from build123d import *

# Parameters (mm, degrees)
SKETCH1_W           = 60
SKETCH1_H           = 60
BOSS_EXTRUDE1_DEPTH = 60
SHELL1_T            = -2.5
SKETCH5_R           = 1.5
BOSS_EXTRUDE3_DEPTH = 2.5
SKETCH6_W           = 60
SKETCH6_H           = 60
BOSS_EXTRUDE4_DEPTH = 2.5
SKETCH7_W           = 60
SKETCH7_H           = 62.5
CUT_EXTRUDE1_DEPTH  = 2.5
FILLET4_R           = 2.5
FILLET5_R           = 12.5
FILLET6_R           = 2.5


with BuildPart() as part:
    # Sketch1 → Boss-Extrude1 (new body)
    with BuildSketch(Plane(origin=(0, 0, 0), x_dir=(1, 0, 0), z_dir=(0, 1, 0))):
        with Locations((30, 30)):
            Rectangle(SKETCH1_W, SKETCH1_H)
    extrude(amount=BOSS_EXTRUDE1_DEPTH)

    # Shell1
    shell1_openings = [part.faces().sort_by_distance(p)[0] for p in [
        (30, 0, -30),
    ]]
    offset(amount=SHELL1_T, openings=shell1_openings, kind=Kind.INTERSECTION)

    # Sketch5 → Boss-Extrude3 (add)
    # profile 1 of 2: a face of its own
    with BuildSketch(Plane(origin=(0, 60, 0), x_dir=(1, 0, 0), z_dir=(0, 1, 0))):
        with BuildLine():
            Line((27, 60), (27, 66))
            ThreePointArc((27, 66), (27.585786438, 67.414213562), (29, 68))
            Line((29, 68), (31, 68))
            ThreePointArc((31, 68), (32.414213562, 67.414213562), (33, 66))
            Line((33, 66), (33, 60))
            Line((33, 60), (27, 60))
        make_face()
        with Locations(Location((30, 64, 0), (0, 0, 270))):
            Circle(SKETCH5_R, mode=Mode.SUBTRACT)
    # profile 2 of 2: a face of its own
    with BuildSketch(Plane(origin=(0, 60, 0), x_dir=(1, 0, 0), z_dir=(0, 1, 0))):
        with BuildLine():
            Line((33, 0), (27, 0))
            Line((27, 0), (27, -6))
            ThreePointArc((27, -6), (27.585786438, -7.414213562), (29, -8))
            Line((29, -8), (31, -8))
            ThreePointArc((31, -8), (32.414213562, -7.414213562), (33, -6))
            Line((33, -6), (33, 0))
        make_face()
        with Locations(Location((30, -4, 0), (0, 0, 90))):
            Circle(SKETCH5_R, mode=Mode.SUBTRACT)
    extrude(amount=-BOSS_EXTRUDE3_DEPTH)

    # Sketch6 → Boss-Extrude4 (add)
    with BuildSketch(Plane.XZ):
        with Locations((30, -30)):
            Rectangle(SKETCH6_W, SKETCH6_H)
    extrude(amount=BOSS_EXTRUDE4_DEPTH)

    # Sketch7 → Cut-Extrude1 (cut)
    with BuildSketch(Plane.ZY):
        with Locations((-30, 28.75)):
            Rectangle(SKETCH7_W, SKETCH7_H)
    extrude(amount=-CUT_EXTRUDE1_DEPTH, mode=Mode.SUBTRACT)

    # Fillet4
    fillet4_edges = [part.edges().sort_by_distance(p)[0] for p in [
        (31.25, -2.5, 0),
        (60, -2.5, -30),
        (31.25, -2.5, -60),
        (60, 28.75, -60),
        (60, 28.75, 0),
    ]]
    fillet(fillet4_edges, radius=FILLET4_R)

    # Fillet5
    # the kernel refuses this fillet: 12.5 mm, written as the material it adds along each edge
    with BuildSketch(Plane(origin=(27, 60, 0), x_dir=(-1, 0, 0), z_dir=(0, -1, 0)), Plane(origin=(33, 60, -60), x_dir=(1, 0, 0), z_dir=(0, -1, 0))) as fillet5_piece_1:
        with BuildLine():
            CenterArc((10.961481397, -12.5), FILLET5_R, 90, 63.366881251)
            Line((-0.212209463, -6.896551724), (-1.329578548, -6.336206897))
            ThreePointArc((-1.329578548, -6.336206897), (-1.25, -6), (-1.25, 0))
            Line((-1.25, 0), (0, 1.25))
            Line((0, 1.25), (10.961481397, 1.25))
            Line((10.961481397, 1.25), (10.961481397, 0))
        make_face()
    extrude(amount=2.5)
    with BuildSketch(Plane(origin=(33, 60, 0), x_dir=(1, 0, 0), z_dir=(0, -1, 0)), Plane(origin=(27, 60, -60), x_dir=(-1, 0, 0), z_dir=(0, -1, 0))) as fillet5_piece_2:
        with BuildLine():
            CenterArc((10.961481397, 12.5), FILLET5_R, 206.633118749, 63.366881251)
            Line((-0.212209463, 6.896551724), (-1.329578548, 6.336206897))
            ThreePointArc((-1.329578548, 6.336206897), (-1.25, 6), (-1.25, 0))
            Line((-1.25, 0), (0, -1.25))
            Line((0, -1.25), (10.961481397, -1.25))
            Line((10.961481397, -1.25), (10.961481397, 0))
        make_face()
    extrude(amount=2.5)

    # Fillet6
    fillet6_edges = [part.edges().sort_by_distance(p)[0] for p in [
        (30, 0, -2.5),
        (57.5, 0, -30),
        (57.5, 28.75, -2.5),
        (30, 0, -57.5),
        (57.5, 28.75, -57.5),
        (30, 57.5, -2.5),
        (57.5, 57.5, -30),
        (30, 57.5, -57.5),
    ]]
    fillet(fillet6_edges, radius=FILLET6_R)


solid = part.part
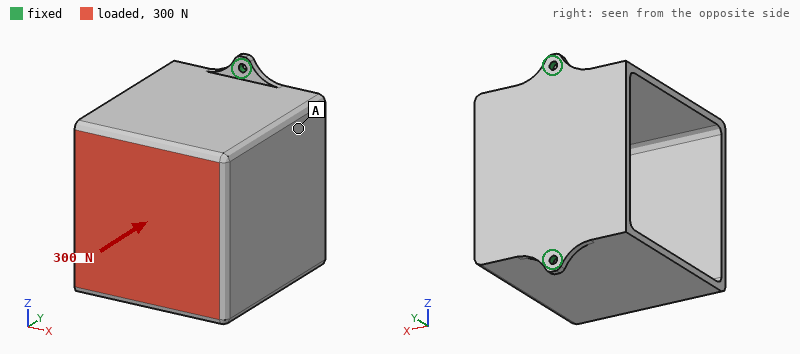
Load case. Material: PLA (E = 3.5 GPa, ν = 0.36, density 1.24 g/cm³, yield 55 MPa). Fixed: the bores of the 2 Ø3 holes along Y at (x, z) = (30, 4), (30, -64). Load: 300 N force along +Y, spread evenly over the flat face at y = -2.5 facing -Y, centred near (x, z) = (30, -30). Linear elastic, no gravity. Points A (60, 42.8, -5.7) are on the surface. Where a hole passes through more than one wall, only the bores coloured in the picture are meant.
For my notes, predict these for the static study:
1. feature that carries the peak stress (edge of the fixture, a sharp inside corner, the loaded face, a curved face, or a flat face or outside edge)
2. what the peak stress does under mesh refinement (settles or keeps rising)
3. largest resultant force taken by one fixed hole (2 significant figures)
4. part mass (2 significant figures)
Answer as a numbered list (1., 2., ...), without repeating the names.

1. edge of the fixture
2. keeps rising
3. 150 N
4. 52 g
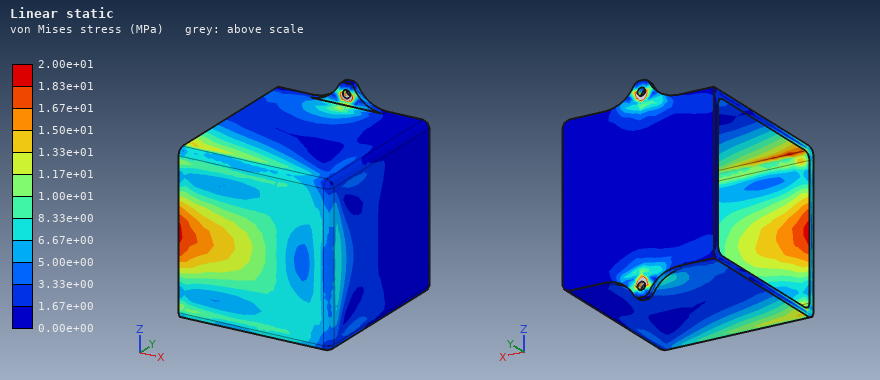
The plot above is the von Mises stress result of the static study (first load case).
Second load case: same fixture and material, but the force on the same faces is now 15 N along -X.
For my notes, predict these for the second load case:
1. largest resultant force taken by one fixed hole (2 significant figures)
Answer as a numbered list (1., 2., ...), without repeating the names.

1. 7.5 N
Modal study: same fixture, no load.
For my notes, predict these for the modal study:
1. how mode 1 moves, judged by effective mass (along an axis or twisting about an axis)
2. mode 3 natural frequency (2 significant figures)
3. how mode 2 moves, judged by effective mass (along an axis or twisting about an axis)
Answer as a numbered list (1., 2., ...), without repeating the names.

1. along X
2. 780 Hz
3. along Z
